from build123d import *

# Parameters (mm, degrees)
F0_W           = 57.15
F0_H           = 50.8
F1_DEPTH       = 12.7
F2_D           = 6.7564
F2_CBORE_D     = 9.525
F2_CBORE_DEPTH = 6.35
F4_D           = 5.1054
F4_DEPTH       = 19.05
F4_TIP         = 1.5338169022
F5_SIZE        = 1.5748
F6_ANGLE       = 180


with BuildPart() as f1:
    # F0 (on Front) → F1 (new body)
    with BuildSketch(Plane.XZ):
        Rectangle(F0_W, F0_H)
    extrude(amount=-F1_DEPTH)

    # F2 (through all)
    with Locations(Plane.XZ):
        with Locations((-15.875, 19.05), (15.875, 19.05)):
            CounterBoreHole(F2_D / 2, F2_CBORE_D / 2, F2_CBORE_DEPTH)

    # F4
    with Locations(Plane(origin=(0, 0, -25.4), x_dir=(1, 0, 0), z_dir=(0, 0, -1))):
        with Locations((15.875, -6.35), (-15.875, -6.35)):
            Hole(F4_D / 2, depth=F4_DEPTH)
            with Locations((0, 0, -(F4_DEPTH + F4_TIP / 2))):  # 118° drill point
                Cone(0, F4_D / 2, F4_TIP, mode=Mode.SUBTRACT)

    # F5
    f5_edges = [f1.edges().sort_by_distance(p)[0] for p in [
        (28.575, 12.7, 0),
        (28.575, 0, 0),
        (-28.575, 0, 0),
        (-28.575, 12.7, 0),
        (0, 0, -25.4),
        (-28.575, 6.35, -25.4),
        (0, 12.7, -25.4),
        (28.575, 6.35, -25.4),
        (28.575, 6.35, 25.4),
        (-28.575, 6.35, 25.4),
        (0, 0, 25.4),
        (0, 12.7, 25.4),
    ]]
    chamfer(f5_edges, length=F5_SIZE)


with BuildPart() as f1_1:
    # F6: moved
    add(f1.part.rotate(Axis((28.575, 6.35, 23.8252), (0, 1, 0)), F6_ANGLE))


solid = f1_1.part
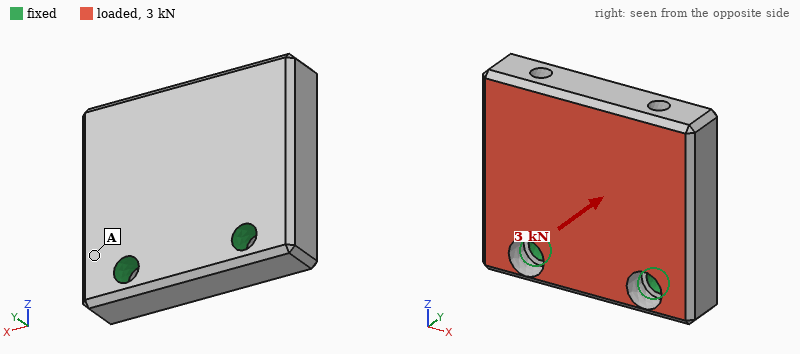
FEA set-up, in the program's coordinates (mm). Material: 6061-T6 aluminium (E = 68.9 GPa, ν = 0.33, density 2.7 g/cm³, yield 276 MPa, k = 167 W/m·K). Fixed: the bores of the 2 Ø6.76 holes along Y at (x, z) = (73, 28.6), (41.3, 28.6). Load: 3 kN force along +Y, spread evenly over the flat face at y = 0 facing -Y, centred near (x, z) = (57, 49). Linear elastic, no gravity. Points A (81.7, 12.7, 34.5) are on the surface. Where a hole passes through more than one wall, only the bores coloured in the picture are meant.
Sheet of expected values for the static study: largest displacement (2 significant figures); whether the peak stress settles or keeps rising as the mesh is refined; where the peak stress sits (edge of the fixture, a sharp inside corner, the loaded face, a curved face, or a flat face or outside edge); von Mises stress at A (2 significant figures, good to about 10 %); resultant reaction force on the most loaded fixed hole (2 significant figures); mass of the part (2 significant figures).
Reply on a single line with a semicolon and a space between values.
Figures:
0.12 mm; keeps rising; edge of the fixture; 32 MPa; 1.5 kN; 92 g
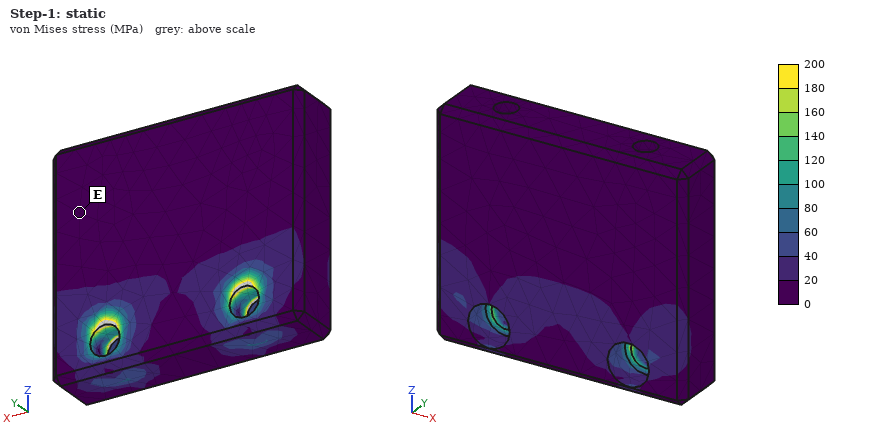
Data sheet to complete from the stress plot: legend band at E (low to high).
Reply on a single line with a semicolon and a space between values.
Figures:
0 to 20 MPa
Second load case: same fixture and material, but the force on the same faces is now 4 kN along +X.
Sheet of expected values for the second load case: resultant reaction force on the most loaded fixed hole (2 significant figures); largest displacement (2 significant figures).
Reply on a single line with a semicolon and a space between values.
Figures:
3.1 kN; 21 µm
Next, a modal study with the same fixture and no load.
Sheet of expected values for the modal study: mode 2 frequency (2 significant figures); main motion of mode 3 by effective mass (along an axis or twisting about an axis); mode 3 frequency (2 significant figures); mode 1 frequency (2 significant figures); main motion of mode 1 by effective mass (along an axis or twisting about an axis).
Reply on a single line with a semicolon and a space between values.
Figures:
7700 Hz; along X; 10 kHz; 3200 Hz; along Y
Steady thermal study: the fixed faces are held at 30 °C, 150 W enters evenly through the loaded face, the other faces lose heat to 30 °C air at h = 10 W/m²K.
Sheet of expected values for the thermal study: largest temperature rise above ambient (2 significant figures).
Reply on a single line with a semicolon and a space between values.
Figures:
35 K
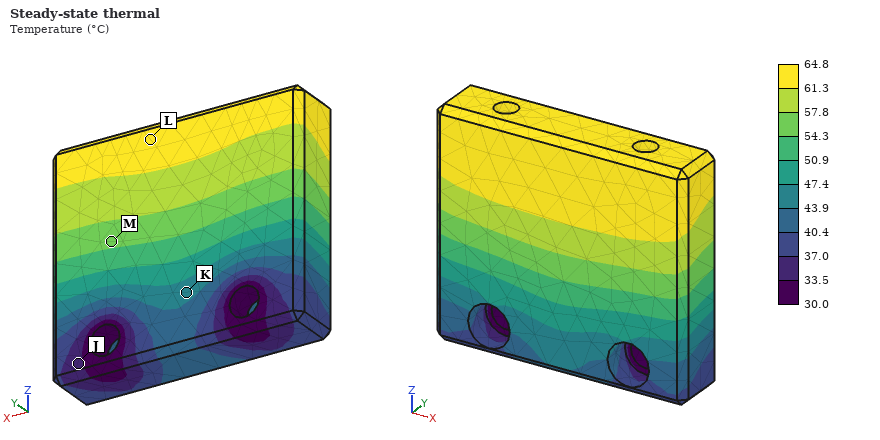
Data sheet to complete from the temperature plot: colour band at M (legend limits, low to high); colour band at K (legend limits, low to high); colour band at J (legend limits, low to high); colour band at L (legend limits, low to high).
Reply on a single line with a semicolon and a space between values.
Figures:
54.3 to 57.8 °C; 43.9 to 47.4 °C; 33.5 to 37.0 °C; 61.3 to 64.8 °C
